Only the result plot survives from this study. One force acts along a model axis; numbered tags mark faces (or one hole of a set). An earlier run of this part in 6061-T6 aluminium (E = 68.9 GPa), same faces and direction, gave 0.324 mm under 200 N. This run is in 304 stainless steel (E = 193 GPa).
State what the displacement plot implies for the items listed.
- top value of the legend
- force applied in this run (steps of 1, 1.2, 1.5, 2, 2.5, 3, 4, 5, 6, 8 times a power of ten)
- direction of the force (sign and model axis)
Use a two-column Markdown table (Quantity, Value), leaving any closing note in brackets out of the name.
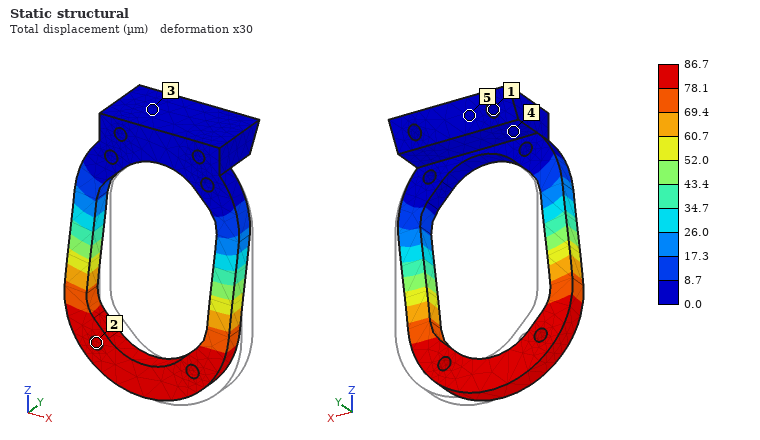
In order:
| Quantity | Value |
|---|---|
| top value of the legend | 86.7 µm |
| force applied in this run | 150 N |
| direction of the force | -X |
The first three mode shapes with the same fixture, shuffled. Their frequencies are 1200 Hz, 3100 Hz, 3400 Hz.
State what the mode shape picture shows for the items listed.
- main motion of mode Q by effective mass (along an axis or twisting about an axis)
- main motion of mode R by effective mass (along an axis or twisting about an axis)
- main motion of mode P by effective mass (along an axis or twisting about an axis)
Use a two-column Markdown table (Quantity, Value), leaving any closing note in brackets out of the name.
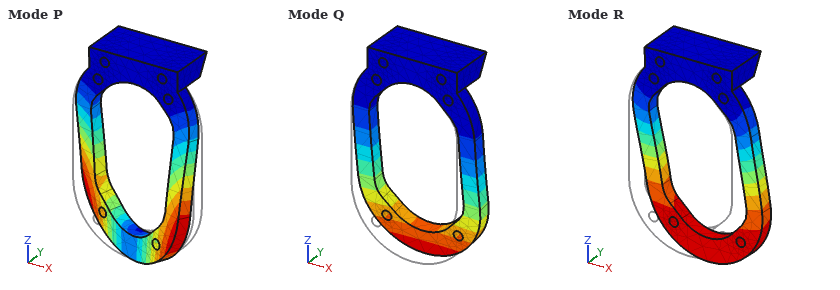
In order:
| Quantity | Value |
|---|---|
| main motion of mode Q by effective mass | along Y |
| main motion of mode R by effective mass | along X |
| main motion of mode P by effective mass | twisting about Z |
